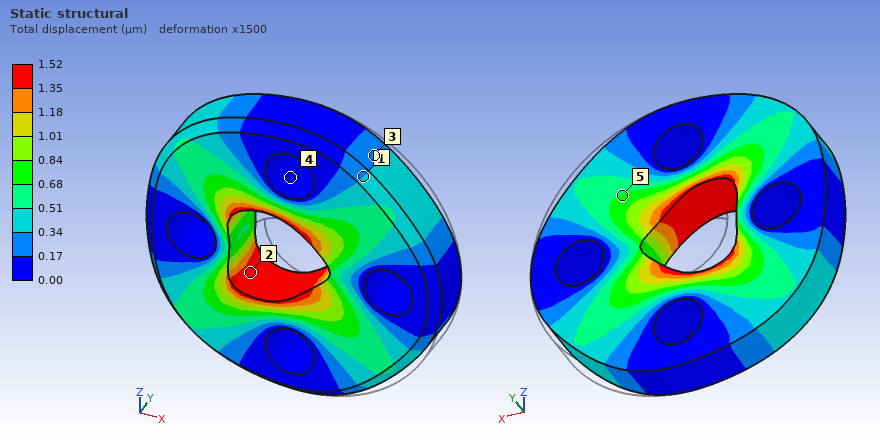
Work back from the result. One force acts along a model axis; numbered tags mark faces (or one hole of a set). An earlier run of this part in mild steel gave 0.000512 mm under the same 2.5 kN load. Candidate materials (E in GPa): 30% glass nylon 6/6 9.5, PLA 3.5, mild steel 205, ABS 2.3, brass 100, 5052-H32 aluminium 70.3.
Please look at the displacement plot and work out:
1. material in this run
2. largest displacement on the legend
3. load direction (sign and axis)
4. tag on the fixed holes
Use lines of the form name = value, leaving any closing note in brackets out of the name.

material in this run = 5052-H32 aluminium
largest displacement on the legend = 1.52 µm
load direction = -X
tag on the fixed holes = 4
